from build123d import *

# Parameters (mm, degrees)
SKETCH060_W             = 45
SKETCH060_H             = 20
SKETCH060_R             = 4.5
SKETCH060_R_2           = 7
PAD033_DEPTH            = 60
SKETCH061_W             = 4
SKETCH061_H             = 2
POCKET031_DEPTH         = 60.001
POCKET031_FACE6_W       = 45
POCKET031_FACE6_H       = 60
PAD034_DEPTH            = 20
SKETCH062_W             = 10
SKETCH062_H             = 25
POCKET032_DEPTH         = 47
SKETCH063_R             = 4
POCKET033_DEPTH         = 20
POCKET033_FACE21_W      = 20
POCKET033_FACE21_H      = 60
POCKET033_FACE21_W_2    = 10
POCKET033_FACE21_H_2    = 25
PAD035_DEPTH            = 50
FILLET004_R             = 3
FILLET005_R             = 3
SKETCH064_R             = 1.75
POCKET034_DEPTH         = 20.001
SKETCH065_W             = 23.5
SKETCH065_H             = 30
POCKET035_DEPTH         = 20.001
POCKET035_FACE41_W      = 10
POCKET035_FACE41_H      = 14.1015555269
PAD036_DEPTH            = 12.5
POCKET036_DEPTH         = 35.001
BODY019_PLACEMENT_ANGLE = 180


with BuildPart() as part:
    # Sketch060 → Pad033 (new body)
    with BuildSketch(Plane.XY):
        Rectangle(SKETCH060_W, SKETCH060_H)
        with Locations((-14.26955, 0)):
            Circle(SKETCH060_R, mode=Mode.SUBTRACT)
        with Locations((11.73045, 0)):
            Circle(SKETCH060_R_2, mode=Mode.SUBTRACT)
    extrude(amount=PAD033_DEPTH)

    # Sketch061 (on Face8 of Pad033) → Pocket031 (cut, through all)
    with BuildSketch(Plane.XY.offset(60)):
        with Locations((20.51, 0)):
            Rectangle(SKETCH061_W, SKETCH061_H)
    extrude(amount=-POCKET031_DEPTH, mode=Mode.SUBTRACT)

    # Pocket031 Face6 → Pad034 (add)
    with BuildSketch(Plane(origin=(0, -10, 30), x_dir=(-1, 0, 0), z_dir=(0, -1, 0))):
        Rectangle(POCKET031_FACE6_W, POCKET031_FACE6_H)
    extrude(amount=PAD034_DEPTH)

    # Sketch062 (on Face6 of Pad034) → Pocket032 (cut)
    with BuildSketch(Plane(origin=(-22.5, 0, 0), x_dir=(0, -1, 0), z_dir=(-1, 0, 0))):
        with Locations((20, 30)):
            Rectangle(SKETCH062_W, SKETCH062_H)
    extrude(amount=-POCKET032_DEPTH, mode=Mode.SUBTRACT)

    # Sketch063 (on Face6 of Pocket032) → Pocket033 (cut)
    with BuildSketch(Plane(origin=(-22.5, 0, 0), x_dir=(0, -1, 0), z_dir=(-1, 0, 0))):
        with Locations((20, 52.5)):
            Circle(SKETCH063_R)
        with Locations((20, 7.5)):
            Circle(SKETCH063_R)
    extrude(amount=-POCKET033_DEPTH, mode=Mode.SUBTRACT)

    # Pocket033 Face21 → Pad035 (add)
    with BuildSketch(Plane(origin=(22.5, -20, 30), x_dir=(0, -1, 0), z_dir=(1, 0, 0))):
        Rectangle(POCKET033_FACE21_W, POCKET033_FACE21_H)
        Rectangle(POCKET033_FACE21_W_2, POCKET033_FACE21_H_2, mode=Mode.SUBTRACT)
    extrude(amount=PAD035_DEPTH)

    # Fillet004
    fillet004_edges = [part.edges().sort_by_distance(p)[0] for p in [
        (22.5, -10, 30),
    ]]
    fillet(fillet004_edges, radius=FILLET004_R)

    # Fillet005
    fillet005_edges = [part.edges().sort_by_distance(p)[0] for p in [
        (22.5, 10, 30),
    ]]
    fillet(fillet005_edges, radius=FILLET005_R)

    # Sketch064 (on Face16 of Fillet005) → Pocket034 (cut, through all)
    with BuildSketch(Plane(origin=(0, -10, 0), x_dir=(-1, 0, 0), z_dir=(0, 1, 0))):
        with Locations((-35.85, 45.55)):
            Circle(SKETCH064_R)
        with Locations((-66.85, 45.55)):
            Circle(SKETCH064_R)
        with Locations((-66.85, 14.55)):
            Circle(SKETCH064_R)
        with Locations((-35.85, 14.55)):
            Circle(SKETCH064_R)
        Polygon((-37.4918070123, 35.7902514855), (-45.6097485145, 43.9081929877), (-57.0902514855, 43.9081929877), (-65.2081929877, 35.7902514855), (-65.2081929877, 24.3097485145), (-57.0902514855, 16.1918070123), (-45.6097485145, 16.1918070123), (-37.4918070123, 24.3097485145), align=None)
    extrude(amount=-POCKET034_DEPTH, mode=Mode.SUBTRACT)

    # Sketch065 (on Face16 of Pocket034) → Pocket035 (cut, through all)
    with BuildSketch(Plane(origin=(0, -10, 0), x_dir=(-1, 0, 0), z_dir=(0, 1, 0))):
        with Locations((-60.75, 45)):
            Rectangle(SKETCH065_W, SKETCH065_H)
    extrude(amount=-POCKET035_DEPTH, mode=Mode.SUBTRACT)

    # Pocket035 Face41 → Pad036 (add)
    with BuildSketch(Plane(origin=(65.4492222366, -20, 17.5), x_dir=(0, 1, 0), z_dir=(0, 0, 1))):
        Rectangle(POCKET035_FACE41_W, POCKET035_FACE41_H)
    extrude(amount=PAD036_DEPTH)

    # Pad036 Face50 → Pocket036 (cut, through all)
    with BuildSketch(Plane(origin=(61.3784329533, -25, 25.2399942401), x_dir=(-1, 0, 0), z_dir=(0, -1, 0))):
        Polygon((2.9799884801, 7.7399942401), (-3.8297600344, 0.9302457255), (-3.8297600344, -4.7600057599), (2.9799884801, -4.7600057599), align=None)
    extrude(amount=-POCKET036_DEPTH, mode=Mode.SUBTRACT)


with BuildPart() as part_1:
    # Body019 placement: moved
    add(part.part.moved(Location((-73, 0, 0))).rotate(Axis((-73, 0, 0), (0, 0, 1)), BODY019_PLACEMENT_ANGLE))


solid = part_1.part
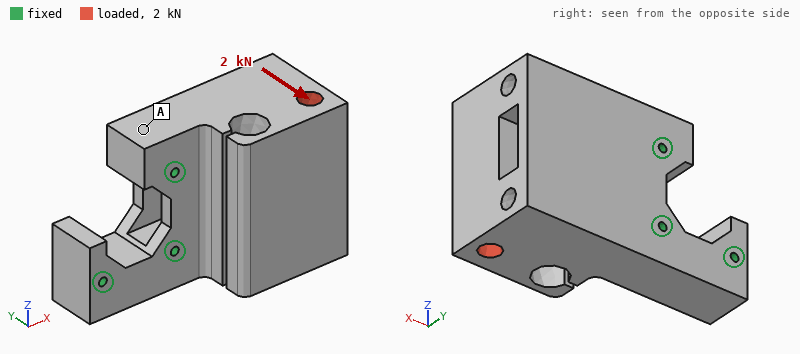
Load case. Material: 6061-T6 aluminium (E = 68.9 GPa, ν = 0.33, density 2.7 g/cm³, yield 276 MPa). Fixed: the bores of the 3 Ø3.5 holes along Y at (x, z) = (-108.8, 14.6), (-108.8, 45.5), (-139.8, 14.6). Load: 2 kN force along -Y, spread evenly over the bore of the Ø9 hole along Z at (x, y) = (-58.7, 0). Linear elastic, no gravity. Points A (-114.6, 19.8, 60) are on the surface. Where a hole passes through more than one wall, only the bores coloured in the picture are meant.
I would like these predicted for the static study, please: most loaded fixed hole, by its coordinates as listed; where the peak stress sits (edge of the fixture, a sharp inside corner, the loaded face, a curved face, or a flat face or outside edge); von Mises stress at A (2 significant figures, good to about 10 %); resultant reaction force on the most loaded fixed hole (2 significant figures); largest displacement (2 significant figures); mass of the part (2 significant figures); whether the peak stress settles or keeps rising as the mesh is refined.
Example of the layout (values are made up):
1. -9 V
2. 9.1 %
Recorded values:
1. (-108.8, 14.6)
2. edge of the fixture
3. 6.8 MPa
4. 1.4 kN
5. 68 µm
6. 310 g
7. keeps rising
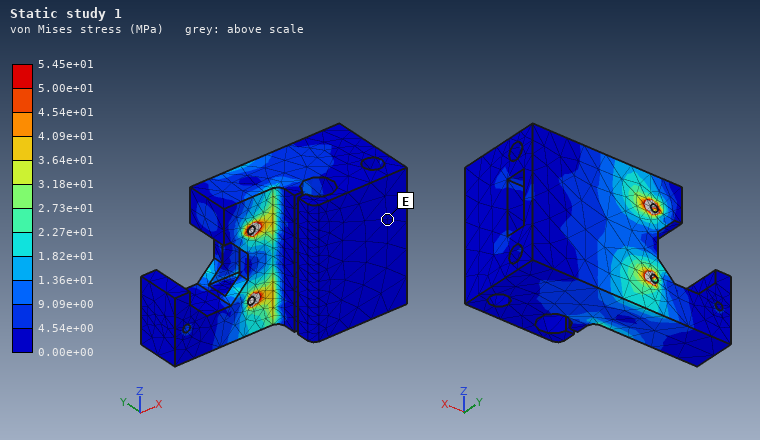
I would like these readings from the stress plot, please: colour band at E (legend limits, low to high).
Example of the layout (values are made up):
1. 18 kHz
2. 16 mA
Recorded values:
1. 0.00e+00 to 4.54e+00 MPa
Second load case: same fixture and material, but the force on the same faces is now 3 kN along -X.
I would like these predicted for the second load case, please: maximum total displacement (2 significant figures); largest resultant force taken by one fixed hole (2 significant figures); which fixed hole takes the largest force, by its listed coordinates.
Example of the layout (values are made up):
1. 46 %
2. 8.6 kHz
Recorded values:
1. 48 µm
2. 1.6 kN
3. (-108.8, 45.5)
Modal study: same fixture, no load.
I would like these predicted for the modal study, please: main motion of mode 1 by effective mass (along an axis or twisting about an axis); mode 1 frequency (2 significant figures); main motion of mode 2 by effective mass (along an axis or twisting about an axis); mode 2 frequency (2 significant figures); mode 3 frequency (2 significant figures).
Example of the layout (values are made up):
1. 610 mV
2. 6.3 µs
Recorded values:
1. along Y
2. 2700 Hz
3. along Z
4. 4800 Hz
5. 6100 Hz
